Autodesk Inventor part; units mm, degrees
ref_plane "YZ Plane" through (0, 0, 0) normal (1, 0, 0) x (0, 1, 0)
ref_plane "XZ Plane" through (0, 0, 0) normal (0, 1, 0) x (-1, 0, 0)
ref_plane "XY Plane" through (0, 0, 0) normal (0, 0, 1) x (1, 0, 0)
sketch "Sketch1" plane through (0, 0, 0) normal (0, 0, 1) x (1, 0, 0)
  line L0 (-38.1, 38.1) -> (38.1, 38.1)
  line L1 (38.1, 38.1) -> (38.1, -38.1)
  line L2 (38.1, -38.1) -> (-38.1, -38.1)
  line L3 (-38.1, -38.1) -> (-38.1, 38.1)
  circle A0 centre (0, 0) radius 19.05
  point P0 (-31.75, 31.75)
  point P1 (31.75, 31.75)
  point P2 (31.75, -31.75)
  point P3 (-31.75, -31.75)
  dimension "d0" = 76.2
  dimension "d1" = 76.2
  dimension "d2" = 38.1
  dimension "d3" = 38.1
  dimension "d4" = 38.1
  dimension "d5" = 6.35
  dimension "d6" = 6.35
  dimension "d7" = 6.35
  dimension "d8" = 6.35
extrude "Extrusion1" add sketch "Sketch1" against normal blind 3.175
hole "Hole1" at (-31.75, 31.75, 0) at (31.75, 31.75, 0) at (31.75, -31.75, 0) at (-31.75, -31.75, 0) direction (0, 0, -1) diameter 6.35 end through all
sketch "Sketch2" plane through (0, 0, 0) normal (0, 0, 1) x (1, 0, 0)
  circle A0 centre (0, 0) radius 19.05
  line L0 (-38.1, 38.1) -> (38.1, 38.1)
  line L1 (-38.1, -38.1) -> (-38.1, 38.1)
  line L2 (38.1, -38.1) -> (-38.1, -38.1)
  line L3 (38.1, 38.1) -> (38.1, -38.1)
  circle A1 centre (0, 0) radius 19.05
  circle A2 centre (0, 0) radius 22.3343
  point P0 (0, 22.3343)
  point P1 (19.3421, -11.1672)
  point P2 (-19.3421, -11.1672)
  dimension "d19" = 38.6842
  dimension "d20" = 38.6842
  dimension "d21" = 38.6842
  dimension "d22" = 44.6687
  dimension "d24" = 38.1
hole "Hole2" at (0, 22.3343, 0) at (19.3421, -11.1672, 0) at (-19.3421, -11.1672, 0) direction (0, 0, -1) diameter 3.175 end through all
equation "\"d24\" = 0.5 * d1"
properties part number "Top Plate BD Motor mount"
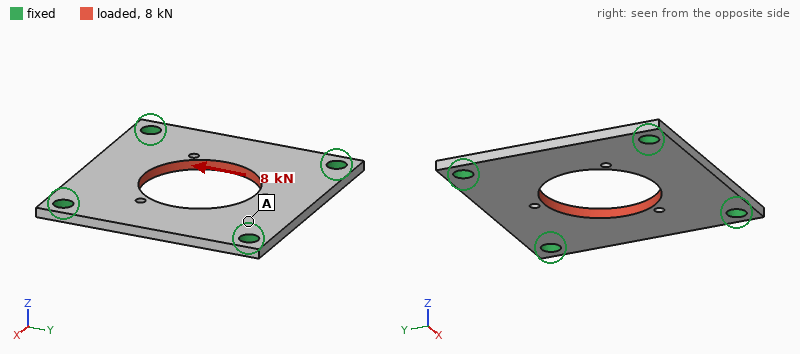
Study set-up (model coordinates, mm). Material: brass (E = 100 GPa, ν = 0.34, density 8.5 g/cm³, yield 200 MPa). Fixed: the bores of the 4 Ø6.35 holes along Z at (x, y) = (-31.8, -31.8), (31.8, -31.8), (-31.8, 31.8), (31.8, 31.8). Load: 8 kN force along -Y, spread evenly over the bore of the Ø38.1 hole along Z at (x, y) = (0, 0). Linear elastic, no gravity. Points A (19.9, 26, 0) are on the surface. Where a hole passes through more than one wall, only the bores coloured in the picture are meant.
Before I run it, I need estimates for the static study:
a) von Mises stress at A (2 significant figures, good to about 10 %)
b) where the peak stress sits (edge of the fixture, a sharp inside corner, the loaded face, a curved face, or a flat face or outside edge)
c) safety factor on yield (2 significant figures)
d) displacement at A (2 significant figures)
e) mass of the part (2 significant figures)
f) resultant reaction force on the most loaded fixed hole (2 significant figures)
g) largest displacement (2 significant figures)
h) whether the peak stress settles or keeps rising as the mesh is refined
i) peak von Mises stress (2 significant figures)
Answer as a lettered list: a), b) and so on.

a) 31 MPa
b) a curved face
c) 1.7
d) 8.4 µm
e) 120 g
f) 2.2 kN
g) 20 µm
h) settles
i) 120 MPa
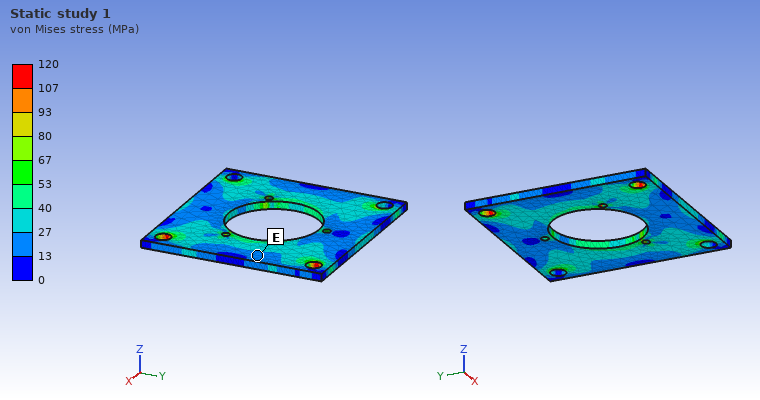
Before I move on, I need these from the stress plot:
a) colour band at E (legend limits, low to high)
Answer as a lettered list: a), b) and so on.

a) 13 to 27 MPa
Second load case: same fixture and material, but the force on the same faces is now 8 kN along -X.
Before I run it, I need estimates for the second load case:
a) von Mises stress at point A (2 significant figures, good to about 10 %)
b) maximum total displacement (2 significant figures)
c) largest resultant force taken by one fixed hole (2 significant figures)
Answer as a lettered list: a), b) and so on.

a) 30 MPa
b) 19 µm
c) 2.2 kN
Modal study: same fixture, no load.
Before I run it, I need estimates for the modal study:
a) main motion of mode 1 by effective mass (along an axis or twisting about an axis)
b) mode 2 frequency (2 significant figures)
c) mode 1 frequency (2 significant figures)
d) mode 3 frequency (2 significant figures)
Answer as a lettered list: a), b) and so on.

a) along Z
b) 3200 Hz
c) 2500 Hz
d) 3200 Hz
